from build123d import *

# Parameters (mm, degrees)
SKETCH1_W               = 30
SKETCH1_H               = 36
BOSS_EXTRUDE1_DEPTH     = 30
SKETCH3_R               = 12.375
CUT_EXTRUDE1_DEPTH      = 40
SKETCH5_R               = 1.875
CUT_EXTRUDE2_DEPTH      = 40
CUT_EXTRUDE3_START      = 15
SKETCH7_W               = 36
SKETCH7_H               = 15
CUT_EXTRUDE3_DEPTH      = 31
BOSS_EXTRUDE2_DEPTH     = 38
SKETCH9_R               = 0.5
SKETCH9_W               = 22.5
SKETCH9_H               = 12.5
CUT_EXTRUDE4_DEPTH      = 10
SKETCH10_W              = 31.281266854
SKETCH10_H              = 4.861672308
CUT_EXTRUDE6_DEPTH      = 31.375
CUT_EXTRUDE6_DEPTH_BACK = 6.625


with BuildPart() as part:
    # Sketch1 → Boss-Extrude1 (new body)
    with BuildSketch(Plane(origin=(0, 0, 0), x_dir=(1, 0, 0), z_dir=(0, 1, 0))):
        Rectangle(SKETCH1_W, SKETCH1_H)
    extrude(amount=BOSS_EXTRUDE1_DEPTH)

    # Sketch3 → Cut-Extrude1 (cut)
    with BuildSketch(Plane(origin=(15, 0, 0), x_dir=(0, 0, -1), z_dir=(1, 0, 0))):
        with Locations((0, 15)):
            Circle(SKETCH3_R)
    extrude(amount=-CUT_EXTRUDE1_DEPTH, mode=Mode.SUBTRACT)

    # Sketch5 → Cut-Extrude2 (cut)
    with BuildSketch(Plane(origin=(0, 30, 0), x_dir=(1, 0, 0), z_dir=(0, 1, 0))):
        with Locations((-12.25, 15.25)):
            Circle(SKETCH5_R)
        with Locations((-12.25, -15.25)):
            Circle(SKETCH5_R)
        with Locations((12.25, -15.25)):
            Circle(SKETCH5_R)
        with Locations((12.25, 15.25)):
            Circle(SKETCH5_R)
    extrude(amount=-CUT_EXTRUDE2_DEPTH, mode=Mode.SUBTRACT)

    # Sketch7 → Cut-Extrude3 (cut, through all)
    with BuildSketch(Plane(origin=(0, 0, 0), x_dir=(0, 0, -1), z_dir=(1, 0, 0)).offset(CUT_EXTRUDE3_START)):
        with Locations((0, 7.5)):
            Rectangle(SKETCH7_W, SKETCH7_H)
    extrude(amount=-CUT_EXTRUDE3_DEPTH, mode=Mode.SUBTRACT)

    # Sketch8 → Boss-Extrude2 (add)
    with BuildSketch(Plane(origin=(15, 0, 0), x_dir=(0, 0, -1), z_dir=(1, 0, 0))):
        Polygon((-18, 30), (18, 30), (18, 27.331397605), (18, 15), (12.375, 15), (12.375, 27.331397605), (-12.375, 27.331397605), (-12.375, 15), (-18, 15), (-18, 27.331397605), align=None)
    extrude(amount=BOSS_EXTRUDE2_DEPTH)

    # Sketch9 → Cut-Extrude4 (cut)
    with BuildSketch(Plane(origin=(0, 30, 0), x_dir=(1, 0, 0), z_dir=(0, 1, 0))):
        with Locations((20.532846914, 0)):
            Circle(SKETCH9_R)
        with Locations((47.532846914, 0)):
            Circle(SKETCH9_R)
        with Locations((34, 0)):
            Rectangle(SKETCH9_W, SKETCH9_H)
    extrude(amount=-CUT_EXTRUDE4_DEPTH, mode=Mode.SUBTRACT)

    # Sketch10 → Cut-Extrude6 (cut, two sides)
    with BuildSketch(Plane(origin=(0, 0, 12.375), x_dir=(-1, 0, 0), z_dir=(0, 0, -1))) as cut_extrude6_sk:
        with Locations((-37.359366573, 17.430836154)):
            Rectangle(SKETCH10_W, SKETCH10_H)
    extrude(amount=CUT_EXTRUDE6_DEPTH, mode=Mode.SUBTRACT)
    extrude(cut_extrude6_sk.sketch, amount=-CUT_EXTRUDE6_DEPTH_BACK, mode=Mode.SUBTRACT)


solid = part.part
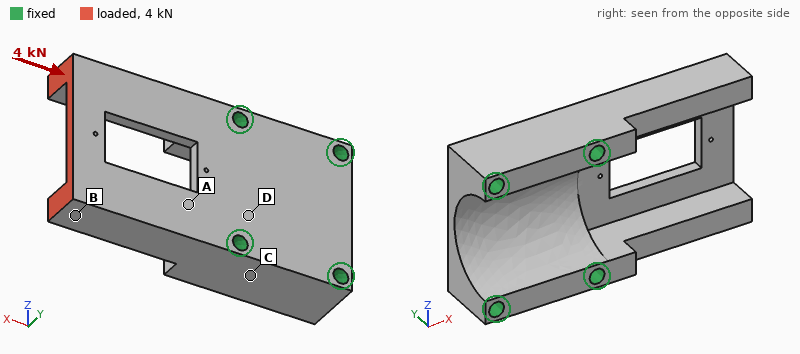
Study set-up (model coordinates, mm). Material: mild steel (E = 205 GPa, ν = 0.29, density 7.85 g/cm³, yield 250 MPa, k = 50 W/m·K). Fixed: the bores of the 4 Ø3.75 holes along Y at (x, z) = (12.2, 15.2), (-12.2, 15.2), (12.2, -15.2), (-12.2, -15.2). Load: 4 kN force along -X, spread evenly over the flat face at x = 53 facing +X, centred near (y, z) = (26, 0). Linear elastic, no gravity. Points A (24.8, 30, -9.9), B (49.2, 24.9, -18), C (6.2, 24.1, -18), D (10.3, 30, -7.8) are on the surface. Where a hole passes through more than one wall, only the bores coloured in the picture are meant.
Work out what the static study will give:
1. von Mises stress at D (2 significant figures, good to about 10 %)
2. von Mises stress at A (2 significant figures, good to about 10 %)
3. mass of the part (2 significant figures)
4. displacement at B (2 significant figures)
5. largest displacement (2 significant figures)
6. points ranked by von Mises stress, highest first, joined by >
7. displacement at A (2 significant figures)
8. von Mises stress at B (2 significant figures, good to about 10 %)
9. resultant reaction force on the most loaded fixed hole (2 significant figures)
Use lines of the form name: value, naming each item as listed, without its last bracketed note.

von Mises stress at D: 9.7 MPa
von Mises stress at A: 34 MPa
mass of the part: 120 g
displacement at B: 6.8 µm
largest displacement: 12 µm
points ranked by von Mises stress, highest first, joined by >: A > B > D > C
displacement at A: 2.5 µm
von Mises stress at B: 20 MPa
resultant reaction force on the most loaded fixed hole: 1.9 kN
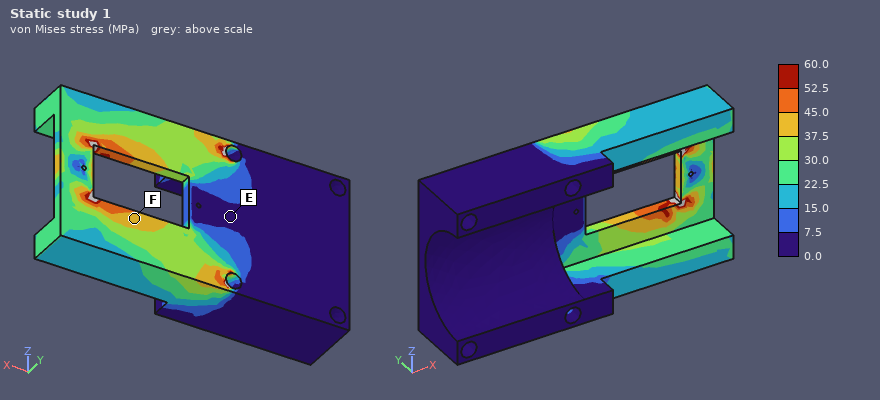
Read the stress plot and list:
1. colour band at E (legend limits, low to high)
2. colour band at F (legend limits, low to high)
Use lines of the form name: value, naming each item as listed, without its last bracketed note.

colour band at E: 0.0 to 7.5 MPa
colour band at F: 37.5 to 45.0 MPa
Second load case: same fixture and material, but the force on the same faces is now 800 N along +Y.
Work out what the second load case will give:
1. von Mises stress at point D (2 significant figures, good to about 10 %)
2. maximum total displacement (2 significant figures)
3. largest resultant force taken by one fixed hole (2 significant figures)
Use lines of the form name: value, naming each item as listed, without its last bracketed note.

von Mises stress at point D: 18 MPa
maximum total displacement: 66 µm
largest resultant force taken by one fixed hole: 540 N
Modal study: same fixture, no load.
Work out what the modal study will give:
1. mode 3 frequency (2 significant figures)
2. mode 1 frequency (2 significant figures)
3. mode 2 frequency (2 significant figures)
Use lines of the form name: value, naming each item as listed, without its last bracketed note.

mode 3 frequency: 8500 Hz
mode 1 frequency: 5600 Hz
mode 2 frequency: 5800 Hz
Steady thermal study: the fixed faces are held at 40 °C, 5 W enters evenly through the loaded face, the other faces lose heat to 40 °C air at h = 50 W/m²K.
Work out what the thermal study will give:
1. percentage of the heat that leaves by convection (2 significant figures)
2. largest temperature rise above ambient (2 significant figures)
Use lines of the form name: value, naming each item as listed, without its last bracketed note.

percentage of the heat that leaves by convection: 35 %
largest temperature rise above ambient: 21 K
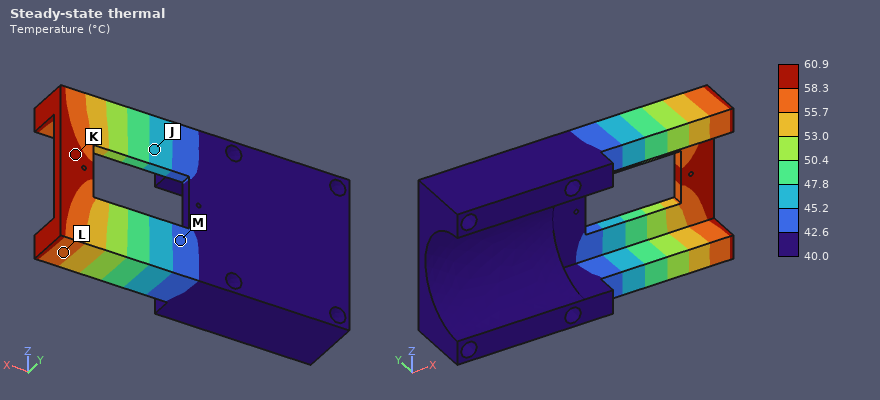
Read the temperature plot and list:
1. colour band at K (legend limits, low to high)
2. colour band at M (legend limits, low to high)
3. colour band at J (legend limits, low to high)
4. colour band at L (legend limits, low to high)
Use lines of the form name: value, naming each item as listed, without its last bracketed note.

colour band at K: 58.3 to 60.9 °C
colour band at M: 42.6 to 45.2 °C
colour band at J: 45.2 to 47.8 °C
colour band at L: 55.7 to 58.3 °C
